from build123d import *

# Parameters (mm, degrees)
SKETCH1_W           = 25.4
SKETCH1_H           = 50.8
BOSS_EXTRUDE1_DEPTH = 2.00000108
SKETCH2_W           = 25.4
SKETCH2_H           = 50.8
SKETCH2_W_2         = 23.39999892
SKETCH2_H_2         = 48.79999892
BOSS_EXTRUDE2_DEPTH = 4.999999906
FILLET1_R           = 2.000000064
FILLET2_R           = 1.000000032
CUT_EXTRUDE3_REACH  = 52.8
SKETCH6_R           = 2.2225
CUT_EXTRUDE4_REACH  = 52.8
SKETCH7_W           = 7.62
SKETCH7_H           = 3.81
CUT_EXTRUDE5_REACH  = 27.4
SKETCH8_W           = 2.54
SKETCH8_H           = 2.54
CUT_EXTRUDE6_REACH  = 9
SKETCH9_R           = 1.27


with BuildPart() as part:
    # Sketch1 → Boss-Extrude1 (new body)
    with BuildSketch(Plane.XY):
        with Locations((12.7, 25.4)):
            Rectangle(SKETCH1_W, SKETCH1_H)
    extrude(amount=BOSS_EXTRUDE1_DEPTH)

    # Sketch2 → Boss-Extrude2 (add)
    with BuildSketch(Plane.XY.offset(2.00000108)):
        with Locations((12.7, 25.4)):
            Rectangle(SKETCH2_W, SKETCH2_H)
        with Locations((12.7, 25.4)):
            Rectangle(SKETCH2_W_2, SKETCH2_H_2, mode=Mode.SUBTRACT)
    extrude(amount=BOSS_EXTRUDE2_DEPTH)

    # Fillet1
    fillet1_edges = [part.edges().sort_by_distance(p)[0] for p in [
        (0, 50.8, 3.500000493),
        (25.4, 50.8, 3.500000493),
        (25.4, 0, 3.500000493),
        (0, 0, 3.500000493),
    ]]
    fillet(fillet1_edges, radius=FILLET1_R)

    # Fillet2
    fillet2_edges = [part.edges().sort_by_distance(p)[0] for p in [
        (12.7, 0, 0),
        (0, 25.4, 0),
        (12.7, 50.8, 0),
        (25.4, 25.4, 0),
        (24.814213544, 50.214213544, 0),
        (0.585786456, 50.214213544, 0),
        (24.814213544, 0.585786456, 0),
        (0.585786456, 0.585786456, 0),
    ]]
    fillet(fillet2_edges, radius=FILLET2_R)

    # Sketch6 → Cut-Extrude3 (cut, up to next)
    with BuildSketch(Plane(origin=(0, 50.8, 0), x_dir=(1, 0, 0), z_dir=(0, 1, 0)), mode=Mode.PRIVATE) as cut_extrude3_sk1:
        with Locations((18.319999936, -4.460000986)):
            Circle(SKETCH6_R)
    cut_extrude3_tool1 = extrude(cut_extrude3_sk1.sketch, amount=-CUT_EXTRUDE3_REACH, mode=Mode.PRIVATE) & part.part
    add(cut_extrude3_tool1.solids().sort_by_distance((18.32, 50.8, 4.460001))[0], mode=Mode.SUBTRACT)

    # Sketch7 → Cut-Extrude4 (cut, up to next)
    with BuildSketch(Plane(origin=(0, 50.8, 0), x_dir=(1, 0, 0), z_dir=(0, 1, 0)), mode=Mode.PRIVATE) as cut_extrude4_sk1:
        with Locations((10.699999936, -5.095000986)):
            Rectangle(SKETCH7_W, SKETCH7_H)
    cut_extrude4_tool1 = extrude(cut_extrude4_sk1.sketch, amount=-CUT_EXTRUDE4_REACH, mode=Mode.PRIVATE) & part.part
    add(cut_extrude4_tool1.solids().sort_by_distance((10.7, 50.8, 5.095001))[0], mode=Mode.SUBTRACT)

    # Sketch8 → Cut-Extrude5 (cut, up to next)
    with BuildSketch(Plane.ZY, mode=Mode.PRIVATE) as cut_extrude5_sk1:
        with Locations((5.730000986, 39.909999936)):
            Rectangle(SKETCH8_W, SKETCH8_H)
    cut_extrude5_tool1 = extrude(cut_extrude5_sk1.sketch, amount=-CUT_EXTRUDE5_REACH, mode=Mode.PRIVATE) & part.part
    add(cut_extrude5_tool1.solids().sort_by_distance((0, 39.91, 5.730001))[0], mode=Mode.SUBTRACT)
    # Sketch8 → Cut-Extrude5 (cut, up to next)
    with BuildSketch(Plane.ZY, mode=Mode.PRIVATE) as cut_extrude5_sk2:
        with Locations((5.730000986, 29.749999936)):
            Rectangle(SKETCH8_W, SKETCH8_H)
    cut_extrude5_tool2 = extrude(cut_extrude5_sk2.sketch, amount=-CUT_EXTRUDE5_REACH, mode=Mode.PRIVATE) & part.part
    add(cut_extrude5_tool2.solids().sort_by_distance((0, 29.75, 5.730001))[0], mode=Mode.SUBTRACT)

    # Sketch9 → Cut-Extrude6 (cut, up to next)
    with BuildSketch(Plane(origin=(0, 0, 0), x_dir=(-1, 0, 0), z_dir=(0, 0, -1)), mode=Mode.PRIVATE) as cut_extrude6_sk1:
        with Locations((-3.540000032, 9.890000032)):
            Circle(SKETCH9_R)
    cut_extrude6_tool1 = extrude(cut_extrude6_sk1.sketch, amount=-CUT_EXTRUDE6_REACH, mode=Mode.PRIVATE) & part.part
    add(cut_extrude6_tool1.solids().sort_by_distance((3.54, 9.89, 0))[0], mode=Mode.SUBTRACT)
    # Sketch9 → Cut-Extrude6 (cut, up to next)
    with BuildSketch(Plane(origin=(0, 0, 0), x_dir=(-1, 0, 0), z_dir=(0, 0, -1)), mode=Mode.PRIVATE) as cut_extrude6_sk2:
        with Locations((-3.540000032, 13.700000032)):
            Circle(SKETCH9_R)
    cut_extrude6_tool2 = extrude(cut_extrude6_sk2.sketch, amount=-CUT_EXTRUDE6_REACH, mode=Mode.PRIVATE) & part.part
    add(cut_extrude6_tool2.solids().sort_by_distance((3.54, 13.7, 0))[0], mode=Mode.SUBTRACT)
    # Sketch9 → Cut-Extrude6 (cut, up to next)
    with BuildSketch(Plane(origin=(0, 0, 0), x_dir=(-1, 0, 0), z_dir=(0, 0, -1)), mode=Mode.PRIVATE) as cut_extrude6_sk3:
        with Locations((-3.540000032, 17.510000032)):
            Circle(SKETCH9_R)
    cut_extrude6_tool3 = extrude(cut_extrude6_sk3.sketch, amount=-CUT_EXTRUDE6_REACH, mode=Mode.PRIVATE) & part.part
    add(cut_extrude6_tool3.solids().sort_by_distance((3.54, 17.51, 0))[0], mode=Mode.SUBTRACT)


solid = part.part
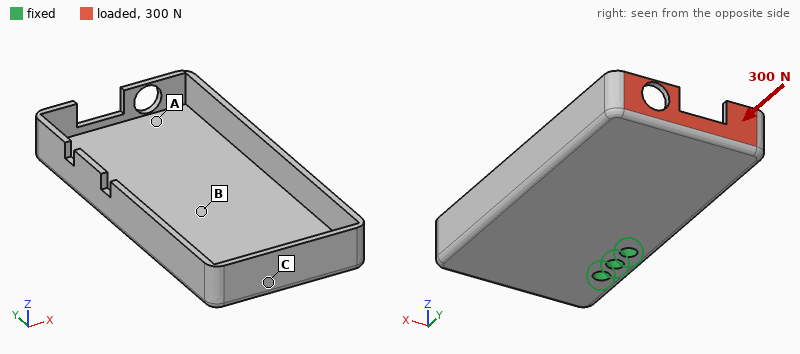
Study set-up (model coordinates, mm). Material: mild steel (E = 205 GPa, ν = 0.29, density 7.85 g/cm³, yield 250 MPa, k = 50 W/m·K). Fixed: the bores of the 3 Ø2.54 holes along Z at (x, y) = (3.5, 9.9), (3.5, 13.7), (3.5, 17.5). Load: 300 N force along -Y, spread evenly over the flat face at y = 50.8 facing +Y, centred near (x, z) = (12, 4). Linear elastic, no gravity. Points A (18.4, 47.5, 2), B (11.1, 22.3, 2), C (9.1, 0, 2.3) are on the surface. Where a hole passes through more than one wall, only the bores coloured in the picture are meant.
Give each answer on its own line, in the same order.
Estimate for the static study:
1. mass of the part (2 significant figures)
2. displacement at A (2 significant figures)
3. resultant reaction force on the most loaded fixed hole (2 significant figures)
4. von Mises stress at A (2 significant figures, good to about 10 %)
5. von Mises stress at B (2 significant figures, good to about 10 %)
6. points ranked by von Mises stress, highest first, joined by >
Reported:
25 g
40 µm
290 N
27 MPa
18 MPa
A > B > C
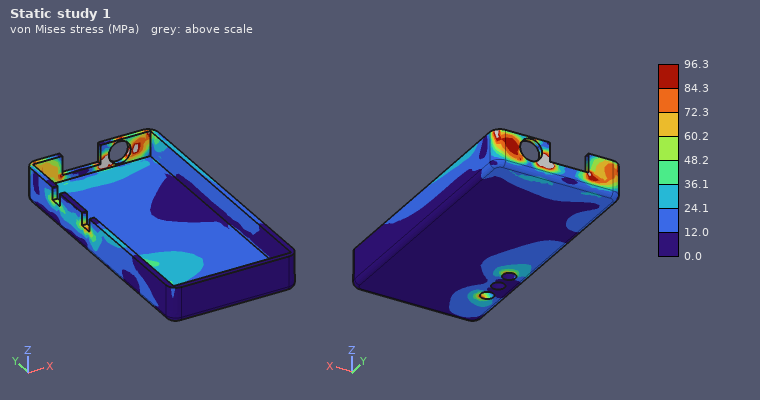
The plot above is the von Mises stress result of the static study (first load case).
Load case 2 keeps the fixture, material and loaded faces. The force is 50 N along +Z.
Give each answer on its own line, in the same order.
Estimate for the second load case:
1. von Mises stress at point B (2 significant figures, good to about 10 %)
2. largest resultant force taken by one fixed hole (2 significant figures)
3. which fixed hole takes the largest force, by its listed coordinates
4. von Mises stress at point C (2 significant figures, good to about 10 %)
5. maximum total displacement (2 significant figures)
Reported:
28 MPa
190 N
(3.5, 17.5)
12 MPa
0.11 mm
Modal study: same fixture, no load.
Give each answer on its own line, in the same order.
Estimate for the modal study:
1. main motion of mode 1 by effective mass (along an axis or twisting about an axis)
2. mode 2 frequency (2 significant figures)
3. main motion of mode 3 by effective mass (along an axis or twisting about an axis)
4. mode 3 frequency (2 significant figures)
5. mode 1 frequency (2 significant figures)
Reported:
along Z
3100 Hz
along Z
4400 Hz
1500 Hz
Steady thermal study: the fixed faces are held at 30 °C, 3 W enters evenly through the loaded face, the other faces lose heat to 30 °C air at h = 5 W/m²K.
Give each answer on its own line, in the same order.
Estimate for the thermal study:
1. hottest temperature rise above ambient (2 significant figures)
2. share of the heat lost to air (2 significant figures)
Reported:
48 K
11 %
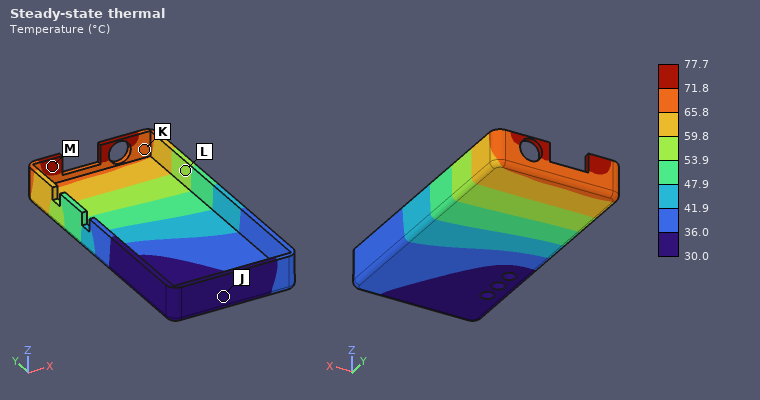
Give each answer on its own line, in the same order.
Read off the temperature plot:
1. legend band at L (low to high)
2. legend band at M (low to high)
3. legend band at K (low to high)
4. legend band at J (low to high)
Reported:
53.9 to 59.8 °C
71.8 to 77.7 °C
65.8 to 71.8 °C
30.0 to 36.0 °C
